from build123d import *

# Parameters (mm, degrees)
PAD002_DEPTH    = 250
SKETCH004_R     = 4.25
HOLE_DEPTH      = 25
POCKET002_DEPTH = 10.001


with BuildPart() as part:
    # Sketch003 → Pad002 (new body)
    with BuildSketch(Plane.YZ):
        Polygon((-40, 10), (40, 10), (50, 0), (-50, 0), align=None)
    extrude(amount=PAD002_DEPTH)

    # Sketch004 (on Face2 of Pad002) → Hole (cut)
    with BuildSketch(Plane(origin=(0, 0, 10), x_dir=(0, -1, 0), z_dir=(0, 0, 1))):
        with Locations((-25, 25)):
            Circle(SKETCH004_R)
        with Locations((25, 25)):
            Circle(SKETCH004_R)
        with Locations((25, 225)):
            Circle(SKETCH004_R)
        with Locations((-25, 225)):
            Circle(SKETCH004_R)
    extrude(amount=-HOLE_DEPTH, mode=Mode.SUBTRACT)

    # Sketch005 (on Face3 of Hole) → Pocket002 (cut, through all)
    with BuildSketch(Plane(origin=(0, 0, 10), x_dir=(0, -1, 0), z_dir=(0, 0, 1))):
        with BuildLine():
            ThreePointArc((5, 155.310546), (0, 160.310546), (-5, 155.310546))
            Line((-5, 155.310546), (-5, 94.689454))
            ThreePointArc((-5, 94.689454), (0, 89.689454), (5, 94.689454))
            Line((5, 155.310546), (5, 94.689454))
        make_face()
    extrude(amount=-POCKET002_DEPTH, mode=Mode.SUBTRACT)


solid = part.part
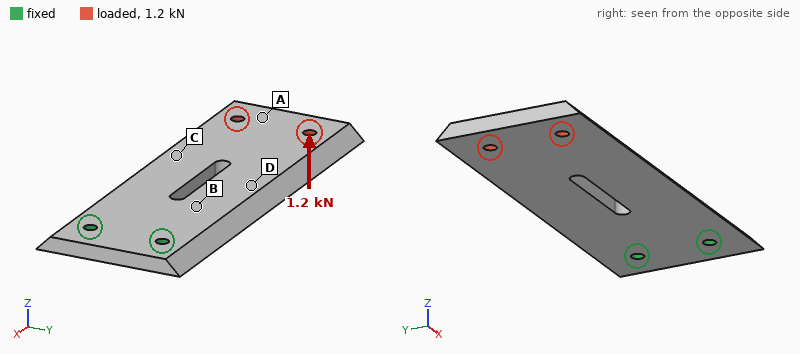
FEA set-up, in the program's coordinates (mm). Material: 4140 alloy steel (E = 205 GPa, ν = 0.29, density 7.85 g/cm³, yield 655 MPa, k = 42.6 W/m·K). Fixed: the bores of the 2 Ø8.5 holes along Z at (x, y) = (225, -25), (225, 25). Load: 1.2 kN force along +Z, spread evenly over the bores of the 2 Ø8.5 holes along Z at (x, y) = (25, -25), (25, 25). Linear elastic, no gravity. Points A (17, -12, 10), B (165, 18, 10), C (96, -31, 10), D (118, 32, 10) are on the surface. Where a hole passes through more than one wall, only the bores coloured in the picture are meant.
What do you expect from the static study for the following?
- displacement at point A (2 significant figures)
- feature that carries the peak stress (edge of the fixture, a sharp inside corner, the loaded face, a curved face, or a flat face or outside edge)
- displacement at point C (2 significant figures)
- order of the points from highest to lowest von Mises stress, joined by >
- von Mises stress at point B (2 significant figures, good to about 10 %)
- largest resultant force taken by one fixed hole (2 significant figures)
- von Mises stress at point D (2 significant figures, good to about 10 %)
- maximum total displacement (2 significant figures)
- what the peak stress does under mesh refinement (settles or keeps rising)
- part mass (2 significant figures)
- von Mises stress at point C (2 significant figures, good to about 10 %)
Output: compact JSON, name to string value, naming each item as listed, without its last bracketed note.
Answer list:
{"displacement at point A": "2.3 mm", "feature that carries the peak stress": "edge of the fixture", "displacement at point C": "1.1 mm", "order of the points from highest to lowest von Mises stress, joined by >": "B > D > C > A", "von Mises stress at point B": "120 MPa", "largest resultant force taken by one fixed hole": "640 N", "von Mises stress at point D": "87 MPa", "maximum total displacement": "2.6 mm", "what the peak stress does under mesh refinement": "keeps rising", "part mass": "1.7 kg", "von Mises stress at point C": "65 MPa"}
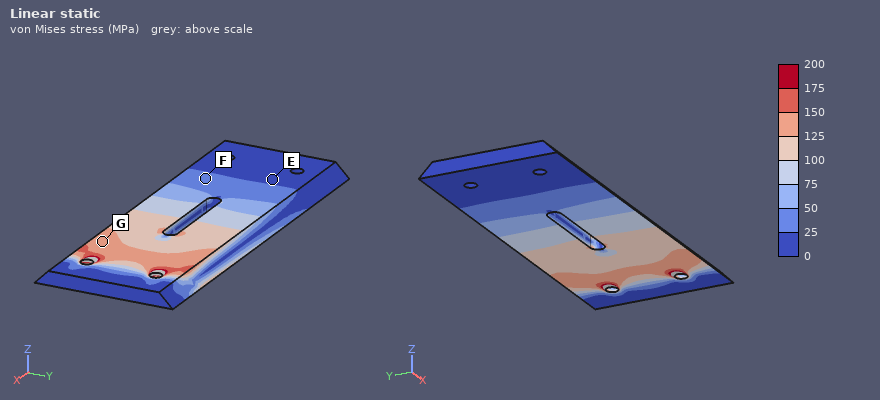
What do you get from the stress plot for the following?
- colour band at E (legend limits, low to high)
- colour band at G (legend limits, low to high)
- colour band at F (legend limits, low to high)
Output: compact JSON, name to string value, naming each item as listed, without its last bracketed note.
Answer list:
{"colour band at E": "0 to 25 MPa", "colour band at G": "125 to 150 MPa", "colour band at F": "25 to 50 MPa"}
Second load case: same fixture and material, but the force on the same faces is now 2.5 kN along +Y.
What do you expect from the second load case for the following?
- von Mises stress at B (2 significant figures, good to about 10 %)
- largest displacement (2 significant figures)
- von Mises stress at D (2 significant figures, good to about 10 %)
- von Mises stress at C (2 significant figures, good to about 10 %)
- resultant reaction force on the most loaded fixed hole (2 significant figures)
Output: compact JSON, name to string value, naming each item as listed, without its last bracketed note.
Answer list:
{"von Mises stress at B": "8.0 MPa", "largest displacement": "92 µm", "von Mises stress at D": "13 MPa", "von Mises stress at C": "7.8 MPa", "resultant reaction force on the most loaded fixed hole": "9.3 kN"}
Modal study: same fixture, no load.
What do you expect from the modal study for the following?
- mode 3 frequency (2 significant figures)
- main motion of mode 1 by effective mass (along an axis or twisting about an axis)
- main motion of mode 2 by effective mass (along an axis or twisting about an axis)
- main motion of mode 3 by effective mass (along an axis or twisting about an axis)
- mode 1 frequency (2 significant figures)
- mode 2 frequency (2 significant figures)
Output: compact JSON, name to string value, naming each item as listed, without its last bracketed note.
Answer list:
{"mode 3 frequency": "1000 Hz", "main motion of mode 1 by effective mass": "along Z", "main motion of mode 2 by effective mass": "twisting about X", "main motion of mode 3 by effective mass": "along Z", "mode 1 frequency": "160 Hz", "mode 2 frequency": "780 Hz"}
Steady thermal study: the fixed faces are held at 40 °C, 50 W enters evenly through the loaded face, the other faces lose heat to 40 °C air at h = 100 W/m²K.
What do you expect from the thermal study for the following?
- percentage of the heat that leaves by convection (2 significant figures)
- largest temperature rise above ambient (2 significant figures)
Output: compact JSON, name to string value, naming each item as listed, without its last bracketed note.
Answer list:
{"percentage of the heat that leaves by convection": "99 %", "largest temperature rise above ambient": "43 K"}
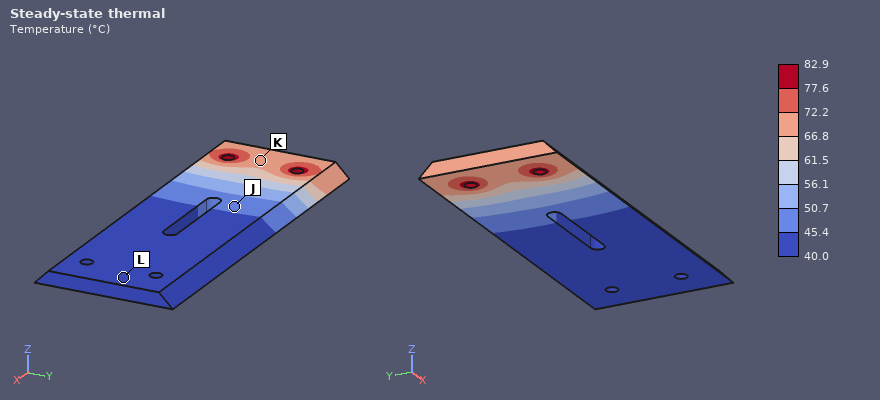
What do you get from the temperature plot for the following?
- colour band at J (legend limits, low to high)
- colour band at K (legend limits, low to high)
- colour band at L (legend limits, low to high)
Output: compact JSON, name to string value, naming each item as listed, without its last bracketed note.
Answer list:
{"colour band at J": "45.4 to 50.7 °C", "colour band at K": "66.8 to 72.2 °C", "colour band at L": "40.0 to 45.4 °C"}
